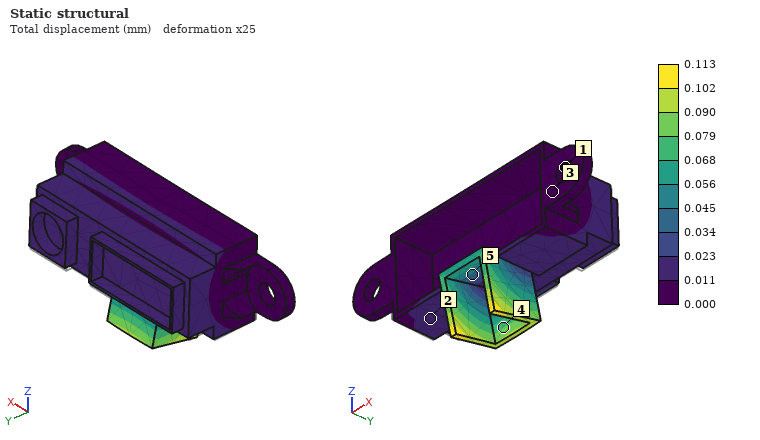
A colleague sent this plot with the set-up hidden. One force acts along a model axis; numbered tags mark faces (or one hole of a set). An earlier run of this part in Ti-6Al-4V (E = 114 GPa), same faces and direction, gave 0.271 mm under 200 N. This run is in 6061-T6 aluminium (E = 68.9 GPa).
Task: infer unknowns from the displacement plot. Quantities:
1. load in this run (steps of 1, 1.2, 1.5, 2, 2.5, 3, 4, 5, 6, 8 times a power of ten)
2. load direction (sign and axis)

50 N
+Y
